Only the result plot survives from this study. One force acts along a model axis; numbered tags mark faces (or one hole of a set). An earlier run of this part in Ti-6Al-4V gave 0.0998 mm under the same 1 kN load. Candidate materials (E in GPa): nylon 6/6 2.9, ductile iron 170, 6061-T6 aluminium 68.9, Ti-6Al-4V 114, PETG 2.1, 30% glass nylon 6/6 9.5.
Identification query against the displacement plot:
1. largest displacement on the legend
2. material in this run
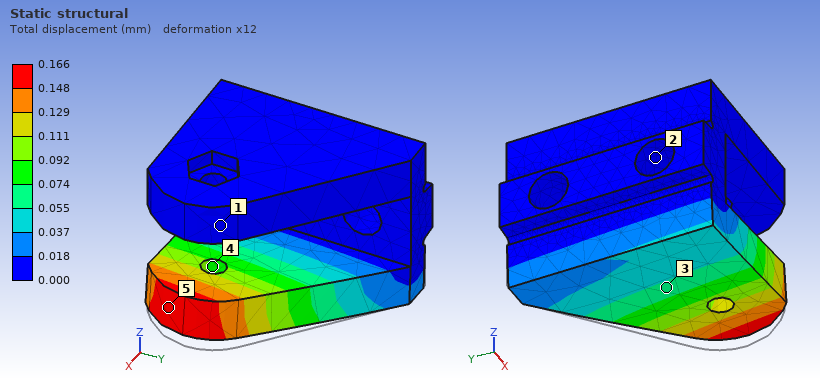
0.166 mm
6061-T6 aluminium
